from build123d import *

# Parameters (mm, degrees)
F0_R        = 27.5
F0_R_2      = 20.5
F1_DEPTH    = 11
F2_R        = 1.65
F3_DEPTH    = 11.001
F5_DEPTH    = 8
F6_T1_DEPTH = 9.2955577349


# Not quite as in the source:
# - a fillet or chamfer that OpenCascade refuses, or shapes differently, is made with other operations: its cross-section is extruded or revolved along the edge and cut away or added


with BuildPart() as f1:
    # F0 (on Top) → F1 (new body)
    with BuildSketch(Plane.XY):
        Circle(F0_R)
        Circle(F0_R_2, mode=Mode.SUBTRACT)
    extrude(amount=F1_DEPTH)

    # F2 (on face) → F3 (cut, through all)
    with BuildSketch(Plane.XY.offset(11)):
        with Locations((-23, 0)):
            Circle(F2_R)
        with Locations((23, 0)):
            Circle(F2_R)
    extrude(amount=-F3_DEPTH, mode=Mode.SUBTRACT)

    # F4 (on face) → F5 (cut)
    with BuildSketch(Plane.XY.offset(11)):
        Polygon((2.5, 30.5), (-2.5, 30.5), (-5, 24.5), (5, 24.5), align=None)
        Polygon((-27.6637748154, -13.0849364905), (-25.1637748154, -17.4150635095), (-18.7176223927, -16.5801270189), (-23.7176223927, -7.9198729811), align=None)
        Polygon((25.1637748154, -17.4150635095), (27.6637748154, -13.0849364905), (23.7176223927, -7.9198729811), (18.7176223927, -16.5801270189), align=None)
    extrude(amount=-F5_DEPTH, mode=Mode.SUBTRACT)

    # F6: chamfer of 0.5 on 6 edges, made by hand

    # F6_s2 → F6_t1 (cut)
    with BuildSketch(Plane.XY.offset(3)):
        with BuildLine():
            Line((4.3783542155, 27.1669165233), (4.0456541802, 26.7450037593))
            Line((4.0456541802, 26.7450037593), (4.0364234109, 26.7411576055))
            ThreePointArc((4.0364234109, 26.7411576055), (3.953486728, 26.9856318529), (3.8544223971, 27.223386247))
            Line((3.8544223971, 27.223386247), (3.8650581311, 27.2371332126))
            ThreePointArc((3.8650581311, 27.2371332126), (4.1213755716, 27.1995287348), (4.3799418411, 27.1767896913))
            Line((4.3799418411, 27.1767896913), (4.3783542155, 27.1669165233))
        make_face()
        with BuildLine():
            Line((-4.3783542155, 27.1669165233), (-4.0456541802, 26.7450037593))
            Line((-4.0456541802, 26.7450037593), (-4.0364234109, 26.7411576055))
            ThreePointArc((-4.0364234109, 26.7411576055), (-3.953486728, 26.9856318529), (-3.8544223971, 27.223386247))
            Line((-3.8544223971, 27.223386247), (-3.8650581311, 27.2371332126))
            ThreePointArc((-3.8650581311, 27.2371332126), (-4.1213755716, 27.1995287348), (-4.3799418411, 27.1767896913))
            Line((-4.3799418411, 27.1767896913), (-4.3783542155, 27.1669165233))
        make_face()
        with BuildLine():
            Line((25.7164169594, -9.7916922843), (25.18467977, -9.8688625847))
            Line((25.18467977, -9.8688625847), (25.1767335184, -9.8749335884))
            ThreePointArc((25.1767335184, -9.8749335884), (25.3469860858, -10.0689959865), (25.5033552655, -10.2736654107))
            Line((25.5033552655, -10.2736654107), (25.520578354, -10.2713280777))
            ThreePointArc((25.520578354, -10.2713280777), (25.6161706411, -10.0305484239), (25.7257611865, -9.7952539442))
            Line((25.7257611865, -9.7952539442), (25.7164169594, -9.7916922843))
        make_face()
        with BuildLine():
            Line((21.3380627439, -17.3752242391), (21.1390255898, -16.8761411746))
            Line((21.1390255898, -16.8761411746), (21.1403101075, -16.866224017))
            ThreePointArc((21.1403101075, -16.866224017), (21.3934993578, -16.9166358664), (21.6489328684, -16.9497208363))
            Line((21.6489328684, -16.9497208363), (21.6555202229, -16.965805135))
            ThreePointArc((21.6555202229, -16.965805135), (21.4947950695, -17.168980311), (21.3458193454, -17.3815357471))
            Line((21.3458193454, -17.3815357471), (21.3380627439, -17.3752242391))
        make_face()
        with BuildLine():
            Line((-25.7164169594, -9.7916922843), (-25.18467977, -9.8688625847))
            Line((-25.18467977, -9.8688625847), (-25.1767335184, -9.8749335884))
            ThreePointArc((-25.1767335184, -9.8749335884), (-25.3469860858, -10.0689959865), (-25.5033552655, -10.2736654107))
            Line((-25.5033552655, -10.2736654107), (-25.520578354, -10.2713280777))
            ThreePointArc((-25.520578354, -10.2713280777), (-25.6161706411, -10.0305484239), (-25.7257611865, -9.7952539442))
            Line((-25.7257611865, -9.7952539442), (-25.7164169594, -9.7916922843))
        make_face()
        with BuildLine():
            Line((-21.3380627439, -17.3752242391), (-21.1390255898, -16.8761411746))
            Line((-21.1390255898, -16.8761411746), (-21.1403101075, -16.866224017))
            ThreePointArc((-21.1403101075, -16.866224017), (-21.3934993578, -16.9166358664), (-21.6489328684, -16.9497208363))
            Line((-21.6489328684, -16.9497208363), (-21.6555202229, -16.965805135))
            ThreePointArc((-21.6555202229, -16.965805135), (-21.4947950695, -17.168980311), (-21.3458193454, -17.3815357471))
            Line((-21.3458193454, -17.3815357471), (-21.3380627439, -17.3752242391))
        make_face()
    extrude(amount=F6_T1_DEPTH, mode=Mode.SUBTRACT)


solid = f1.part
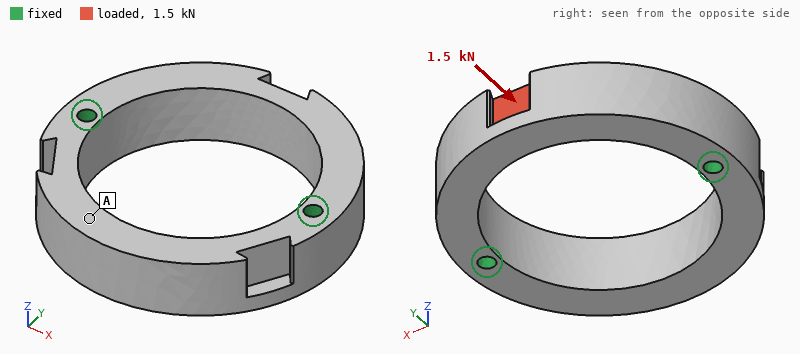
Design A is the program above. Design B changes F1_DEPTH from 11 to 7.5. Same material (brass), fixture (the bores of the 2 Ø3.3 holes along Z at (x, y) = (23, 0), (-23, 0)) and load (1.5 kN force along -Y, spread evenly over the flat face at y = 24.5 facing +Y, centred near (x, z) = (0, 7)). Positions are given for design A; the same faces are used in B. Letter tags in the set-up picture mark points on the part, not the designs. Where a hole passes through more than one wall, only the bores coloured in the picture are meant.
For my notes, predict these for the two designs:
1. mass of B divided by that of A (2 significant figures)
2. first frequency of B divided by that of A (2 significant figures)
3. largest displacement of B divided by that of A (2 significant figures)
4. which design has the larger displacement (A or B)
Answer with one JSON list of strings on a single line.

["0.69", "0.74", "1.4", "B"]
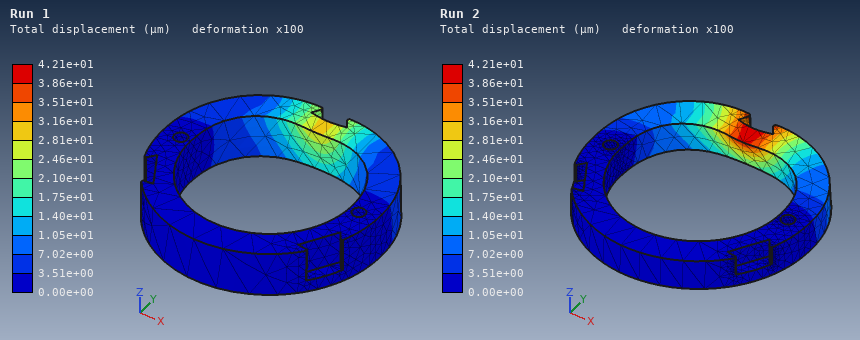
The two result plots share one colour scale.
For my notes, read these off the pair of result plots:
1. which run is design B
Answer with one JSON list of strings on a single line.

["Run 2"]
